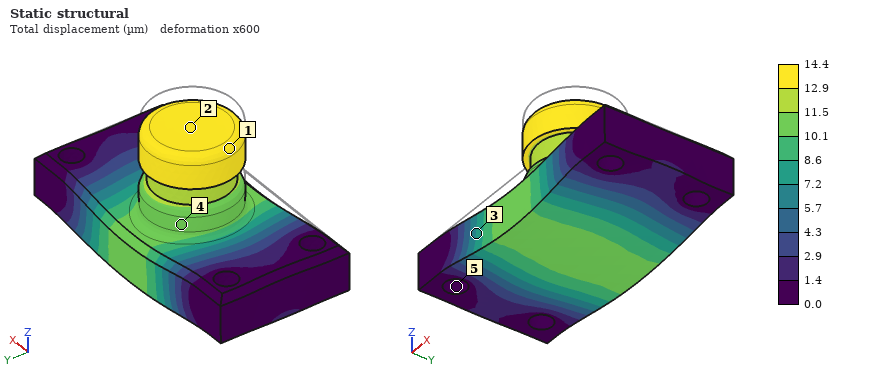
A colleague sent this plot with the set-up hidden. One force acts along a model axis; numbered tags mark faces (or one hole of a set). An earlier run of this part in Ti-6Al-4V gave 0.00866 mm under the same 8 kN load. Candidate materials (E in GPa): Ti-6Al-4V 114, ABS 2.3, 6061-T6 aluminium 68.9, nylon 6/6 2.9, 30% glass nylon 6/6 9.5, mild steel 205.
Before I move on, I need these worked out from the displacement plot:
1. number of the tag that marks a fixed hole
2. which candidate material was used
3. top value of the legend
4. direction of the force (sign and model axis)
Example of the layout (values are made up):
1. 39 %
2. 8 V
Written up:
1. 5
2. 6061-T6 aluminium
3. 14.4 µm
4. -Z
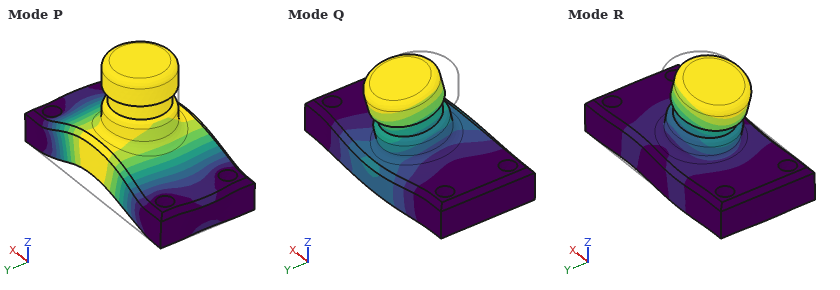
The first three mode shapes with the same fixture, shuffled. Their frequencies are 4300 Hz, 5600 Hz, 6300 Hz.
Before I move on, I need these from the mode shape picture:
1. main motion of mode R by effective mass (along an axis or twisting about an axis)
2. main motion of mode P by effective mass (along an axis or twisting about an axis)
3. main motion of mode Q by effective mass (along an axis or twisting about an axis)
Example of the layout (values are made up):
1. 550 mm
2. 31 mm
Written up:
1. along X
2. along Z
3. along Y
